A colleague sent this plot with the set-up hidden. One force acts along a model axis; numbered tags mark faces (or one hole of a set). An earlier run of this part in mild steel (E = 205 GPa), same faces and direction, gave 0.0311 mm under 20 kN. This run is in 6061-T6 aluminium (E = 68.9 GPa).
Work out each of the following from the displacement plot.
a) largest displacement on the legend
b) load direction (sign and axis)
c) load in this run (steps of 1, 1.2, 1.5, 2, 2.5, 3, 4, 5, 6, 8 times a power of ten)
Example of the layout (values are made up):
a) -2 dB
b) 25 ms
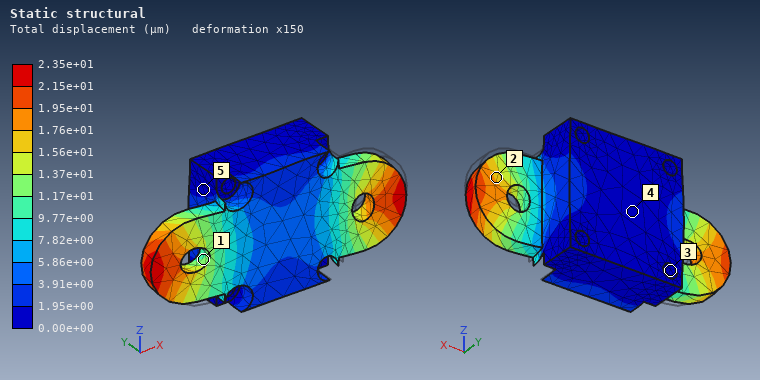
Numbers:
a) 2.35e+01 µm
b) -X
c) 5 kN
